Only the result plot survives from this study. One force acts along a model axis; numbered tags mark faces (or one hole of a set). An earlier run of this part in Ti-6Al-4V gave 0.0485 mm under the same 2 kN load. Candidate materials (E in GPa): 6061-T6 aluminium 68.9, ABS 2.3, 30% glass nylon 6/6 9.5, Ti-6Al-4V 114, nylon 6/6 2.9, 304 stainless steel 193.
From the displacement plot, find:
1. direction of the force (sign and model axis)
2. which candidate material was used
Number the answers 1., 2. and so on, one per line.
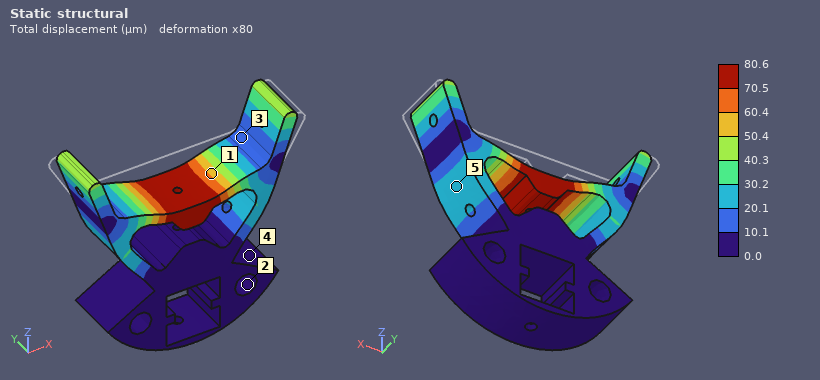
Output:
1. -Z
2. 6061-T6 aluminium
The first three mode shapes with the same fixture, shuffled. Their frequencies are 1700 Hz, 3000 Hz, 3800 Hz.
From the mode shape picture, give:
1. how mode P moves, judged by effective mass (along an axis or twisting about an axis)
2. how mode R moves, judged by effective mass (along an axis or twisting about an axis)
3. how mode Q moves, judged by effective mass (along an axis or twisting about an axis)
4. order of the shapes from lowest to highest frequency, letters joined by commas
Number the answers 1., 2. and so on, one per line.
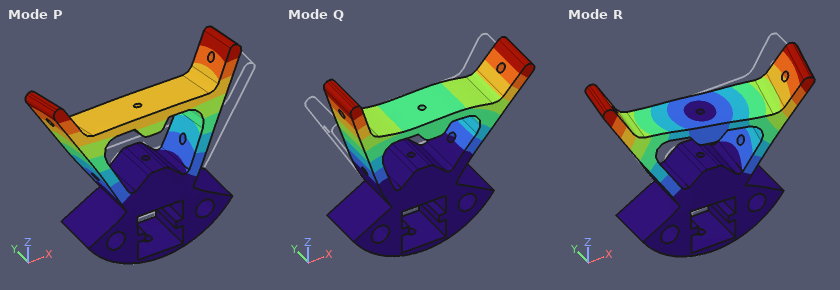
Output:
1. along Y
2. twisting about Z
3. along X
4. Q, P, R
